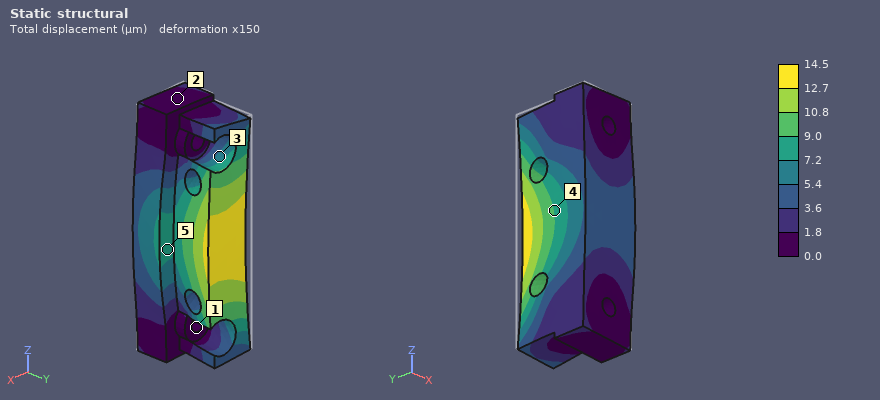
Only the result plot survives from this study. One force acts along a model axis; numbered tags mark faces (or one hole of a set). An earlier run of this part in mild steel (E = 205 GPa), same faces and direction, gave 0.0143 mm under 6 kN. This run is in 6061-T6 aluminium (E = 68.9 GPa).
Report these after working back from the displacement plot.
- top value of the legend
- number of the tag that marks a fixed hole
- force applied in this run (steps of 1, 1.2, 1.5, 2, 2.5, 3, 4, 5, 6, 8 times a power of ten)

14.5 µm
1
2 kN
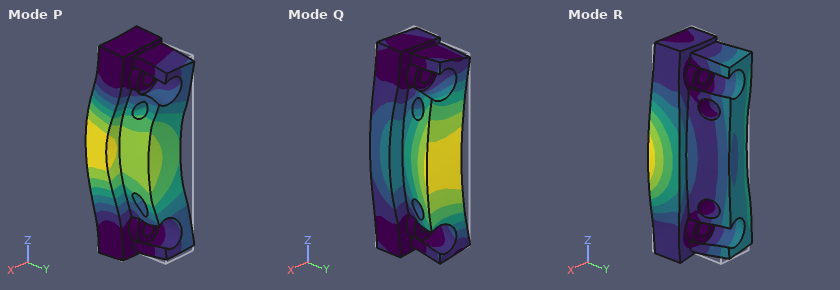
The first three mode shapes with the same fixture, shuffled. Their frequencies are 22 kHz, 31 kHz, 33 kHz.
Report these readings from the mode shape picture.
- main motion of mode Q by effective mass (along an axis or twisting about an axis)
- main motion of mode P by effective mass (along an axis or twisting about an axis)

along X
along Y
